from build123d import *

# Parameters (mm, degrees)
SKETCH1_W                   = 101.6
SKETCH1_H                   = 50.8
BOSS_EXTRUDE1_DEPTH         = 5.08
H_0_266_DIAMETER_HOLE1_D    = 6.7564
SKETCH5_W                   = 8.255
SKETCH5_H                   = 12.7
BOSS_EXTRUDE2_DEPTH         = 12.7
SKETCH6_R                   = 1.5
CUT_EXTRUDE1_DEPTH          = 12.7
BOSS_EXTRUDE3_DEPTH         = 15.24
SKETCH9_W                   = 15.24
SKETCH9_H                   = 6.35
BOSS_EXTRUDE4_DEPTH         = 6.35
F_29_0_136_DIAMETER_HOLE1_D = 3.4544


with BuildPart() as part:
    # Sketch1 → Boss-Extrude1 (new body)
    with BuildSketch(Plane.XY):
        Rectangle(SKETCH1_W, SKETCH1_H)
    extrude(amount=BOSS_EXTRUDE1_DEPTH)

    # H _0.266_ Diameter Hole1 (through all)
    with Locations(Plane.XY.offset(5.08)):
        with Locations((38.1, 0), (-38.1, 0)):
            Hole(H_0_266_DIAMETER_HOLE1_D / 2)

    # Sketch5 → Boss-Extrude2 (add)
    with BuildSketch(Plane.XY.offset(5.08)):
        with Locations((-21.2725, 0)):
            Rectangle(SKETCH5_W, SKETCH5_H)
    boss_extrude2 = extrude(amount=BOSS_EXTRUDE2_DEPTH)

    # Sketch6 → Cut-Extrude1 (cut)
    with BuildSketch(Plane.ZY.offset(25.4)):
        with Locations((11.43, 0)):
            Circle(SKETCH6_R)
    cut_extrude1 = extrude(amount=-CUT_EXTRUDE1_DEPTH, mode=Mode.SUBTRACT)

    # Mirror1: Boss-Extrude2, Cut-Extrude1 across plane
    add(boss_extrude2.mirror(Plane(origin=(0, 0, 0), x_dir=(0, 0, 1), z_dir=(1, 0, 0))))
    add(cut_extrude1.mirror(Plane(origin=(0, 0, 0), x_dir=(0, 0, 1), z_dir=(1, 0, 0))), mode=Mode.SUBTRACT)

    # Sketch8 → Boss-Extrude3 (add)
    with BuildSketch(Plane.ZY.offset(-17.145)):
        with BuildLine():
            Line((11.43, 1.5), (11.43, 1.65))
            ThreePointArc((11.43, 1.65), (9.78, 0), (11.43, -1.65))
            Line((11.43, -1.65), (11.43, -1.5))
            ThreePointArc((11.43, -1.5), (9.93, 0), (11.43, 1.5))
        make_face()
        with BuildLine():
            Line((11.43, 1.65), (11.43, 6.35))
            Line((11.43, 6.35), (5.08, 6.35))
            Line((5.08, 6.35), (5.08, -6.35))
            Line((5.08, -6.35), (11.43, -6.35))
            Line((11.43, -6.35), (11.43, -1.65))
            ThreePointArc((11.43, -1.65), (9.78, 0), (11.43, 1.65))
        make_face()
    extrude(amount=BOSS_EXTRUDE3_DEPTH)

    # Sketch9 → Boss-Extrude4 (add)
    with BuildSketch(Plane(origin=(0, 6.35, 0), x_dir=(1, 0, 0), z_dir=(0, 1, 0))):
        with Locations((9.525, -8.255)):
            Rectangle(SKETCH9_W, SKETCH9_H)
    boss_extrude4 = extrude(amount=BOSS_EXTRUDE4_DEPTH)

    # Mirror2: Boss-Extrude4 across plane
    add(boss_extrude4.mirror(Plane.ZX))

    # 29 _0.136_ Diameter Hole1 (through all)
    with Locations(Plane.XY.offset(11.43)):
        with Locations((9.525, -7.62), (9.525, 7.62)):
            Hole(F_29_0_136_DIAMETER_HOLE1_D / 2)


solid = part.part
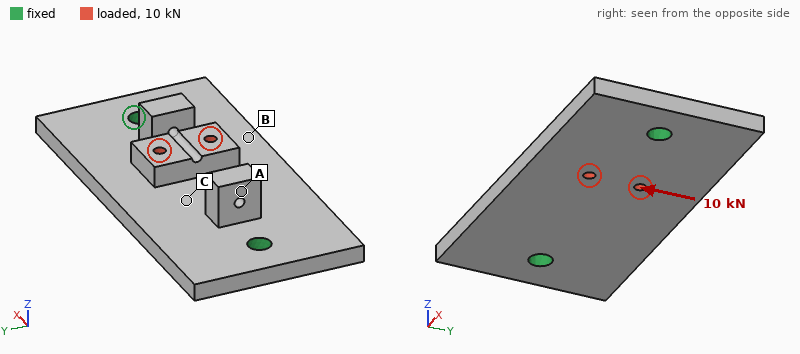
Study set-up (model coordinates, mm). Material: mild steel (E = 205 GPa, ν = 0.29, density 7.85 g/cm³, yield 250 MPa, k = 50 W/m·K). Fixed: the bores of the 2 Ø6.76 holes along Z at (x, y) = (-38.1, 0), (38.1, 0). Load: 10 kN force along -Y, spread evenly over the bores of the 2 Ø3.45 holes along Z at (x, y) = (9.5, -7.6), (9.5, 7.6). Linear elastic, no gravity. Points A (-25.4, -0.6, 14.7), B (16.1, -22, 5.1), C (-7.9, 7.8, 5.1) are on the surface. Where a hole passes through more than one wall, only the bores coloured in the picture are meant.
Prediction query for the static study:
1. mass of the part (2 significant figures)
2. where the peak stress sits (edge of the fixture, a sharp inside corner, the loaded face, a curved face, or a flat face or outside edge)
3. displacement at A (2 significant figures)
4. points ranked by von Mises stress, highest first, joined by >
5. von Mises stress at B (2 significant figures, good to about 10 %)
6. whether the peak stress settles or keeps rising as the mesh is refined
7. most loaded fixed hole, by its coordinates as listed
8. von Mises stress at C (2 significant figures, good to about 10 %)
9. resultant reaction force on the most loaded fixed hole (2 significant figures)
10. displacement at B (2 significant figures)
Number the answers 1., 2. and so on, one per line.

1. 240 g
2. edge of the fixture
3. 19 µm
4. C > B > A
5. 31 MPa
6. keeps rising
7. (38.1, 0)
8. 61 MPa
9. 6.3 kN
10. 47 µm
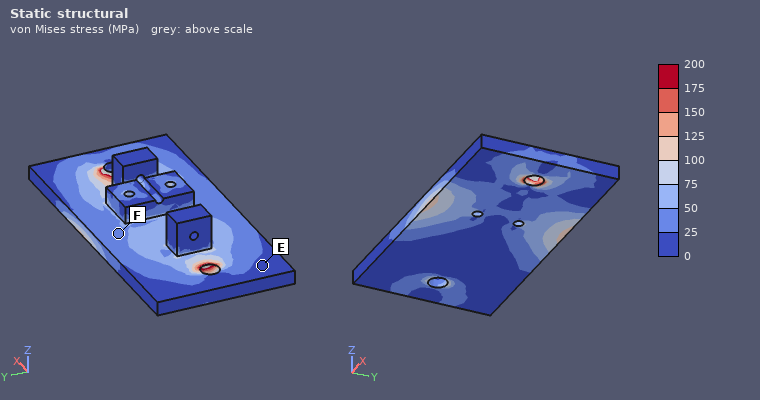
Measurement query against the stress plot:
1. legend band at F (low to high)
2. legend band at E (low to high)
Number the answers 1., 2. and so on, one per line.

1. 25 to 50 MPa
2. 0 to 25 MPa
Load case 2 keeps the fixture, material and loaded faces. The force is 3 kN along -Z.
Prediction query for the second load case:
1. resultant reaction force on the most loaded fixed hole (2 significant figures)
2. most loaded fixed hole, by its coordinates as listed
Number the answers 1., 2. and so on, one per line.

1. 2.0 kN
2. (38.1, 0)
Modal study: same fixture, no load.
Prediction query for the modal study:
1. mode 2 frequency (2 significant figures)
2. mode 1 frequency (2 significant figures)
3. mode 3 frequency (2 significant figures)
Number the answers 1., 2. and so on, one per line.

1. 3800 Hz
2. 3700 Hz
3. 7100 Hz
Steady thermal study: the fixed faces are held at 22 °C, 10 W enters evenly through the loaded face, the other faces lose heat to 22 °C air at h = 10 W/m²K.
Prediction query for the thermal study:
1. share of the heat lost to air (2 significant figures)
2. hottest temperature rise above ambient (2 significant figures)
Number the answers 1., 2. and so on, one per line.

1. 9.6 %
2. 17 K
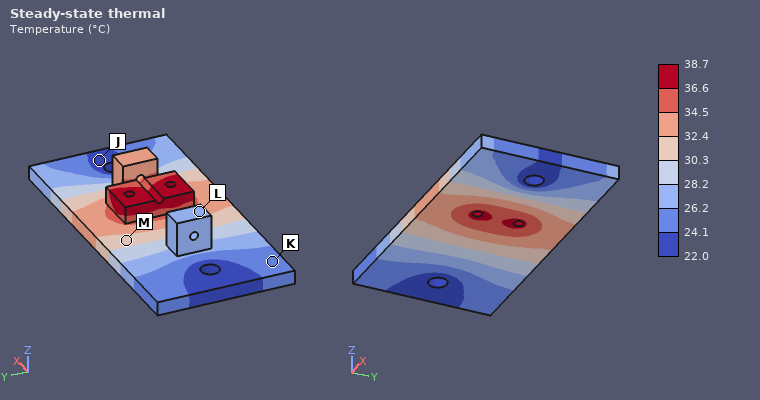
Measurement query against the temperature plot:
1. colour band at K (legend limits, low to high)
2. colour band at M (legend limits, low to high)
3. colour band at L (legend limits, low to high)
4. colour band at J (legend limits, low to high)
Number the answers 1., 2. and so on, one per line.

1. 24.1 to 26.2 °C
2. 30.3 to 32.4 °C
3. 26.2 to 28.2 °C
4. 22.0 to 24.1 °C
